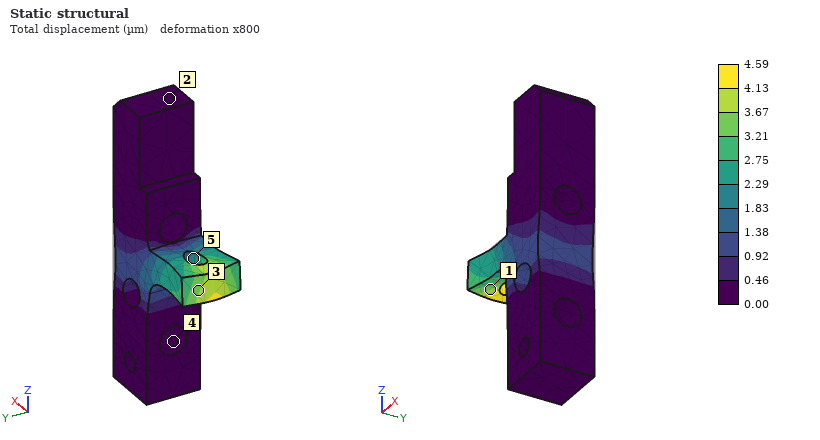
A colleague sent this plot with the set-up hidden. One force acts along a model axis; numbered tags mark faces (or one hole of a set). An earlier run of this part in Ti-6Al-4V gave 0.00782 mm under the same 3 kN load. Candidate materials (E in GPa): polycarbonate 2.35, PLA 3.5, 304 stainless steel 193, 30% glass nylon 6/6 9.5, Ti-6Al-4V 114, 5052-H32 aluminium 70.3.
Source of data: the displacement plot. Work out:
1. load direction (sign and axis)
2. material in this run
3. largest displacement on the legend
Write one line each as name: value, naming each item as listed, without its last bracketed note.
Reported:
load direction: -X
material in this run: 304 stainless steel
largest displacement on the legend: 4.59 µm
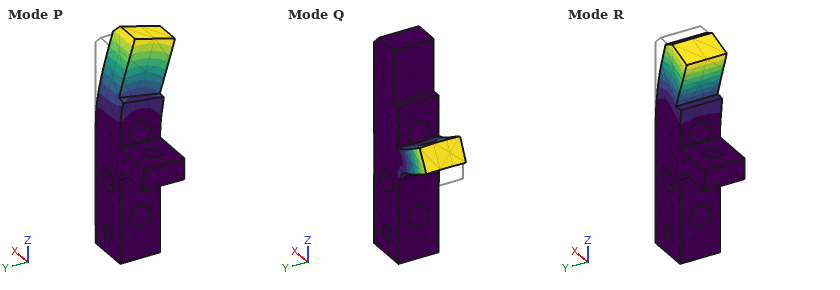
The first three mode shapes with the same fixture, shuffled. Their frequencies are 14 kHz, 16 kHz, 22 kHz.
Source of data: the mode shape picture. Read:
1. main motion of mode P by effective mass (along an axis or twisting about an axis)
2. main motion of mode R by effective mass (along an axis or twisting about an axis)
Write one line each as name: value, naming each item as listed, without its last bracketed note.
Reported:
main motion of mode P by effective mass: along Y
main motion of mode R by effective mass: along X
